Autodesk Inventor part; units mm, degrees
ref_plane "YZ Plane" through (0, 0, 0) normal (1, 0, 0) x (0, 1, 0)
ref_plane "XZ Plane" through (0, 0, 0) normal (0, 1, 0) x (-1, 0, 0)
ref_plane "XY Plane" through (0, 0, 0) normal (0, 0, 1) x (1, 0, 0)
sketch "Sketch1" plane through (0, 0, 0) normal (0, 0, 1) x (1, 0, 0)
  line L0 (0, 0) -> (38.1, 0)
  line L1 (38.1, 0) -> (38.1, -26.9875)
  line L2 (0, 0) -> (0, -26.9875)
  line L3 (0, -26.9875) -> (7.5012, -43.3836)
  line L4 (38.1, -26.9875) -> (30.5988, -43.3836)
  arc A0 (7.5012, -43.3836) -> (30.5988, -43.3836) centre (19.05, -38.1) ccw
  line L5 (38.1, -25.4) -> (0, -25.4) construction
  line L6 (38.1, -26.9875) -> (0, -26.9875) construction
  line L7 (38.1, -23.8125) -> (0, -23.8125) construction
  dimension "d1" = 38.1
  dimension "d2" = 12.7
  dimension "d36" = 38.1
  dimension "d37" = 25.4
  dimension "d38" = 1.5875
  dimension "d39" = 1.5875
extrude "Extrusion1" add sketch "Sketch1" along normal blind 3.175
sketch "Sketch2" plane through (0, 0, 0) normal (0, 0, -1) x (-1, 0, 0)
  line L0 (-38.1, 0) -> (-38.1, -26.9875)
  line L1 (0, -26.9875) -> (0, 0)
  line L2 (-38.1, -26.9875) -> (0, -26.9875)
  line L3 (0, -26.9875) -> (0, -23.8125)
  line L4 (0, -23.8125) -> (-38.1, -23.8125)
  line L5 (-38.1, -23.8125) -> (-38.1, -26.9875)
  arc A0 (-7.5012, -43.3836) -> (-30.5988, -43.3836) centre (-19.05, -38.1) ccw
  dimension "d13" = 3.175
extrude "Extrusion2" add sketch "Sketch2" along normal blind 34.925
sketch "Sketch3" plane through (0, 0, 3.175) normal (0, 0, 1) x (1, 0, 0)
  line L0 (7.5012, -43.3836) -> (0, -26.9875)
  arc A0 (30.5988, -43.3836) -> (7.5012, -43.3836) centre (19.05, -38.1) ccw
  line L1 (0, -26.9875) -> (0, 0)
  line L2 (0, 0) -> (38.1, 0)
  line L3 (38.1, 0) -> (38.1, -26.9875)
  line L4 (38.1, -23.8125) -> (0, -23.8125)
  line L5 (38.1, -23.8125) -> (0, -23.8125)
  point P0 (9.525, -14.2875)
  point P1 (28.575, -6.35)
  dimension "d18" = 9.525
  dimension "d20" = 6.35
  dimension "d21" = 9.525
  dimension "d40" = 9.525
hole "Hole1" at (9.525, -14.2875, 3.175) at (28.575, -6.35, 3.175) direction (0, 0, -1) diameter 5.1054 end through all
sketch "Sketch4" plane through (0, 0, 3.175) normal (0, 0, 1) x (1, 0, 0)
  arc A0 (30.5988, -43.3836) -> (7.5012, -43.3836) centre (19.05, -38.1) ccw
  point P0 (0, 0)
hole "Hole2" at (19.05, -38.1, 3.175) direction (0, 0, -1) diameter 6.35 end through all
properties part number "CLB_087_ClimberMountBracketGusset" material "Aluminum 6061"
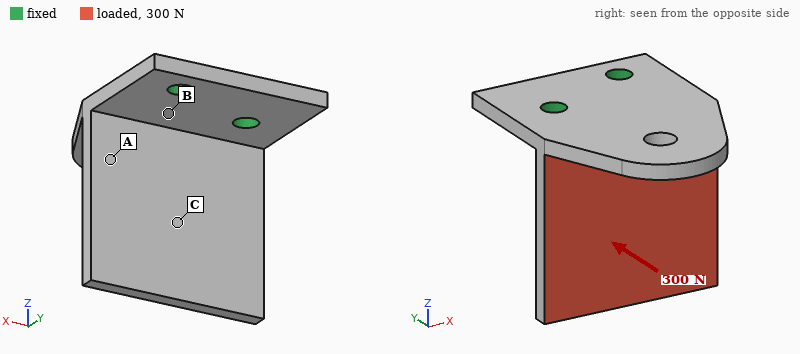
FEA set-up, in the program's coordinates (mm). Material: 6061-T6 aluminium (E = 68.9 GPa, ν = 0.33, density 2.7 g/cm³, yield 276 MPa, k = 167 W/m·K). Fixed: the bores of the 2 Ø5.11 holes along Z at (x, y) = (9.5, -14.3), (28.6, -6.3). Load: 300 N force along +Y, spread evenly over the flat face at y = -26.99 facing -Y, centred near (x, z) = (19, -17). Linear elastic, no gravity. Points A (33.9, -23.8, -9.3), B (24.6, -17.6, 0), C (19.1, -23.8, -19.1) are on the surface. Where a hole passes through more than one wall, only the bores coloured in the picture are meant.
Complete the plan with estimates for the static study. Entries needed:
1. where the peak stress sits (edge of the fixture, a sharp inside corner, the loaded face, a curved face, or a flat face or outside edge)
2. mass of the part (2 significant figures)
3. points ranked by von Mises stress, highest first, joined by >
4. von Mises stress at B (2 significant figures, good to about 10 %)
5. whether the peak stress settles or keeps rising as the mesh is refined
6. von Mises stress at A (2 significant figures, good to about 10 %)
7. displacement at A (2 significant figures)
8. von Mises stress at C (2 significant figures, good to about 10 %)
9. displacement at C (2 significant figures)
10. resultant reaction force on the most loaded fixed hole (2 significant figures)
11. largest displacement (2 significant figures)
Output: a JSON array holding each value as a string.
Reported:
["edge of the fixture", "25 g", "B > A > C", "66 MPa", "keeps rising", "40 MPa", "0.14 mm", "15 MPa", "0.29 mm", "170 N", "0.58 mm"]
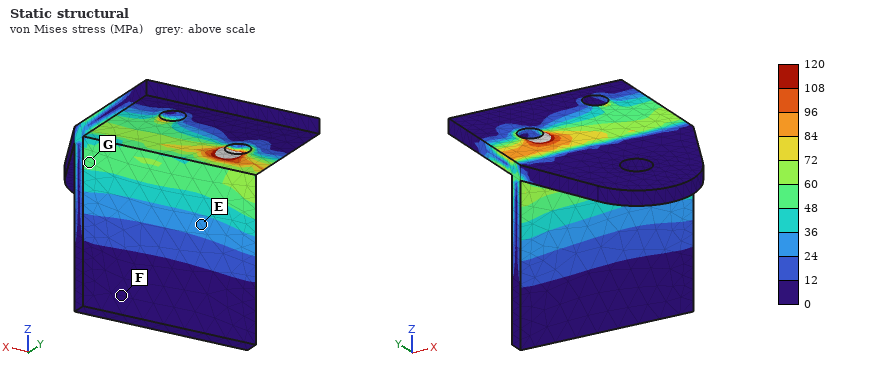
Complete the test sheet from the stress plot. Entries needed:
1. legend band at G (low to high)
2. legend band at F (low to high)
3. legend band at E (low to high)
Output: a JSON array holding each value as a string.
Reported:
["48 to 60 MPa", "0 to 12 MPa", "24 to 36 MPa"]
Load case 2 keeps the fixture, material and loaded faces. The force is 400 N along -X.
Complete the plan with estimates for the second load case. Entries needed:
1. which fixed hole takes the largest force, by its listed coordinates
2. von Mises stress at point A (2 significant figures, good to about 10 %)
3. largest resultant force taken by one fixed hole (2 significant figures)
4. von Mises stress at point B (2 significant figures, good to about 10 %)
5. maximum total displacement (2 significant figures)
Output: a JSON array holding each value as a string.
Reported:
["(9.5, -14.3)", "13 MPa", "480 N", "39 MPa", "0.17 mm"]
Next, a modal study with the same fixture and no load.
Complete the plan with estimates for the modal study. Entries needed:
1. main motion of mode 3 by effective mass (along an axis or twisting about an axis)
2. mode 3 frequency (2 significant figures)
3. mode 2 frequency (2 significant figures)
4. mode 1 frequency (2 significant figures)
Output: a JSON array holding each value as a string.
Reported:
["along Z", "3700 Hz", "2600 Hz", "1200 Hz"]
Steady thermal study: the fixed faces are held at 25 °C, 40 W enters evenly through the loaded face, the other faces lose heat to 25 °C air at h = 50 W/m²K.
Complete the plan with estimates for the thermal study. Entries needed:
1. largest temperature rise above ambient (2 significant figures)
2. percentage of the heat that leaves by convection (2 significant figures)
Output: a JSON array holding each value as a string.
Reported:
["55 K", "16 %"]
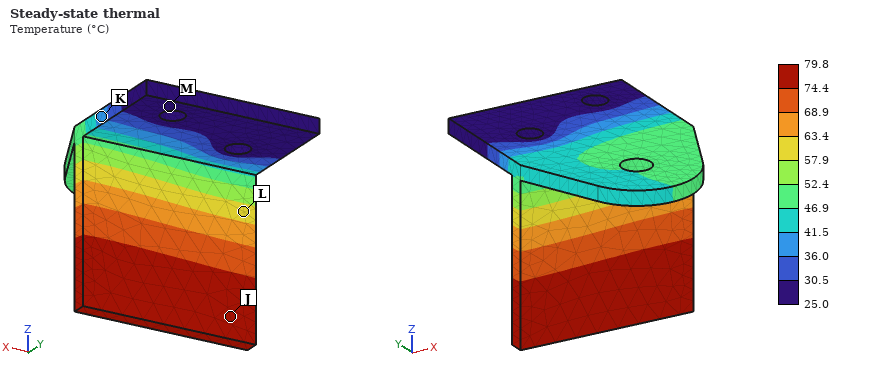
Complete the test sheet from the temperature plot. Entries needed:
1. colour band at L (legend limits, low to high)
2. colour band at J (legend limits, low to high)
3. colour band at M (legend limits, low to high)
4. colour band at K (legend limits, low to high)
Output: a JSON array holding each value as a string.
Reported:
["57.9 to 63.4 °C", "74.4 to 79.8 °C", "25.0 to 30.5 °C", "36.0 to 41.5 °C"]
